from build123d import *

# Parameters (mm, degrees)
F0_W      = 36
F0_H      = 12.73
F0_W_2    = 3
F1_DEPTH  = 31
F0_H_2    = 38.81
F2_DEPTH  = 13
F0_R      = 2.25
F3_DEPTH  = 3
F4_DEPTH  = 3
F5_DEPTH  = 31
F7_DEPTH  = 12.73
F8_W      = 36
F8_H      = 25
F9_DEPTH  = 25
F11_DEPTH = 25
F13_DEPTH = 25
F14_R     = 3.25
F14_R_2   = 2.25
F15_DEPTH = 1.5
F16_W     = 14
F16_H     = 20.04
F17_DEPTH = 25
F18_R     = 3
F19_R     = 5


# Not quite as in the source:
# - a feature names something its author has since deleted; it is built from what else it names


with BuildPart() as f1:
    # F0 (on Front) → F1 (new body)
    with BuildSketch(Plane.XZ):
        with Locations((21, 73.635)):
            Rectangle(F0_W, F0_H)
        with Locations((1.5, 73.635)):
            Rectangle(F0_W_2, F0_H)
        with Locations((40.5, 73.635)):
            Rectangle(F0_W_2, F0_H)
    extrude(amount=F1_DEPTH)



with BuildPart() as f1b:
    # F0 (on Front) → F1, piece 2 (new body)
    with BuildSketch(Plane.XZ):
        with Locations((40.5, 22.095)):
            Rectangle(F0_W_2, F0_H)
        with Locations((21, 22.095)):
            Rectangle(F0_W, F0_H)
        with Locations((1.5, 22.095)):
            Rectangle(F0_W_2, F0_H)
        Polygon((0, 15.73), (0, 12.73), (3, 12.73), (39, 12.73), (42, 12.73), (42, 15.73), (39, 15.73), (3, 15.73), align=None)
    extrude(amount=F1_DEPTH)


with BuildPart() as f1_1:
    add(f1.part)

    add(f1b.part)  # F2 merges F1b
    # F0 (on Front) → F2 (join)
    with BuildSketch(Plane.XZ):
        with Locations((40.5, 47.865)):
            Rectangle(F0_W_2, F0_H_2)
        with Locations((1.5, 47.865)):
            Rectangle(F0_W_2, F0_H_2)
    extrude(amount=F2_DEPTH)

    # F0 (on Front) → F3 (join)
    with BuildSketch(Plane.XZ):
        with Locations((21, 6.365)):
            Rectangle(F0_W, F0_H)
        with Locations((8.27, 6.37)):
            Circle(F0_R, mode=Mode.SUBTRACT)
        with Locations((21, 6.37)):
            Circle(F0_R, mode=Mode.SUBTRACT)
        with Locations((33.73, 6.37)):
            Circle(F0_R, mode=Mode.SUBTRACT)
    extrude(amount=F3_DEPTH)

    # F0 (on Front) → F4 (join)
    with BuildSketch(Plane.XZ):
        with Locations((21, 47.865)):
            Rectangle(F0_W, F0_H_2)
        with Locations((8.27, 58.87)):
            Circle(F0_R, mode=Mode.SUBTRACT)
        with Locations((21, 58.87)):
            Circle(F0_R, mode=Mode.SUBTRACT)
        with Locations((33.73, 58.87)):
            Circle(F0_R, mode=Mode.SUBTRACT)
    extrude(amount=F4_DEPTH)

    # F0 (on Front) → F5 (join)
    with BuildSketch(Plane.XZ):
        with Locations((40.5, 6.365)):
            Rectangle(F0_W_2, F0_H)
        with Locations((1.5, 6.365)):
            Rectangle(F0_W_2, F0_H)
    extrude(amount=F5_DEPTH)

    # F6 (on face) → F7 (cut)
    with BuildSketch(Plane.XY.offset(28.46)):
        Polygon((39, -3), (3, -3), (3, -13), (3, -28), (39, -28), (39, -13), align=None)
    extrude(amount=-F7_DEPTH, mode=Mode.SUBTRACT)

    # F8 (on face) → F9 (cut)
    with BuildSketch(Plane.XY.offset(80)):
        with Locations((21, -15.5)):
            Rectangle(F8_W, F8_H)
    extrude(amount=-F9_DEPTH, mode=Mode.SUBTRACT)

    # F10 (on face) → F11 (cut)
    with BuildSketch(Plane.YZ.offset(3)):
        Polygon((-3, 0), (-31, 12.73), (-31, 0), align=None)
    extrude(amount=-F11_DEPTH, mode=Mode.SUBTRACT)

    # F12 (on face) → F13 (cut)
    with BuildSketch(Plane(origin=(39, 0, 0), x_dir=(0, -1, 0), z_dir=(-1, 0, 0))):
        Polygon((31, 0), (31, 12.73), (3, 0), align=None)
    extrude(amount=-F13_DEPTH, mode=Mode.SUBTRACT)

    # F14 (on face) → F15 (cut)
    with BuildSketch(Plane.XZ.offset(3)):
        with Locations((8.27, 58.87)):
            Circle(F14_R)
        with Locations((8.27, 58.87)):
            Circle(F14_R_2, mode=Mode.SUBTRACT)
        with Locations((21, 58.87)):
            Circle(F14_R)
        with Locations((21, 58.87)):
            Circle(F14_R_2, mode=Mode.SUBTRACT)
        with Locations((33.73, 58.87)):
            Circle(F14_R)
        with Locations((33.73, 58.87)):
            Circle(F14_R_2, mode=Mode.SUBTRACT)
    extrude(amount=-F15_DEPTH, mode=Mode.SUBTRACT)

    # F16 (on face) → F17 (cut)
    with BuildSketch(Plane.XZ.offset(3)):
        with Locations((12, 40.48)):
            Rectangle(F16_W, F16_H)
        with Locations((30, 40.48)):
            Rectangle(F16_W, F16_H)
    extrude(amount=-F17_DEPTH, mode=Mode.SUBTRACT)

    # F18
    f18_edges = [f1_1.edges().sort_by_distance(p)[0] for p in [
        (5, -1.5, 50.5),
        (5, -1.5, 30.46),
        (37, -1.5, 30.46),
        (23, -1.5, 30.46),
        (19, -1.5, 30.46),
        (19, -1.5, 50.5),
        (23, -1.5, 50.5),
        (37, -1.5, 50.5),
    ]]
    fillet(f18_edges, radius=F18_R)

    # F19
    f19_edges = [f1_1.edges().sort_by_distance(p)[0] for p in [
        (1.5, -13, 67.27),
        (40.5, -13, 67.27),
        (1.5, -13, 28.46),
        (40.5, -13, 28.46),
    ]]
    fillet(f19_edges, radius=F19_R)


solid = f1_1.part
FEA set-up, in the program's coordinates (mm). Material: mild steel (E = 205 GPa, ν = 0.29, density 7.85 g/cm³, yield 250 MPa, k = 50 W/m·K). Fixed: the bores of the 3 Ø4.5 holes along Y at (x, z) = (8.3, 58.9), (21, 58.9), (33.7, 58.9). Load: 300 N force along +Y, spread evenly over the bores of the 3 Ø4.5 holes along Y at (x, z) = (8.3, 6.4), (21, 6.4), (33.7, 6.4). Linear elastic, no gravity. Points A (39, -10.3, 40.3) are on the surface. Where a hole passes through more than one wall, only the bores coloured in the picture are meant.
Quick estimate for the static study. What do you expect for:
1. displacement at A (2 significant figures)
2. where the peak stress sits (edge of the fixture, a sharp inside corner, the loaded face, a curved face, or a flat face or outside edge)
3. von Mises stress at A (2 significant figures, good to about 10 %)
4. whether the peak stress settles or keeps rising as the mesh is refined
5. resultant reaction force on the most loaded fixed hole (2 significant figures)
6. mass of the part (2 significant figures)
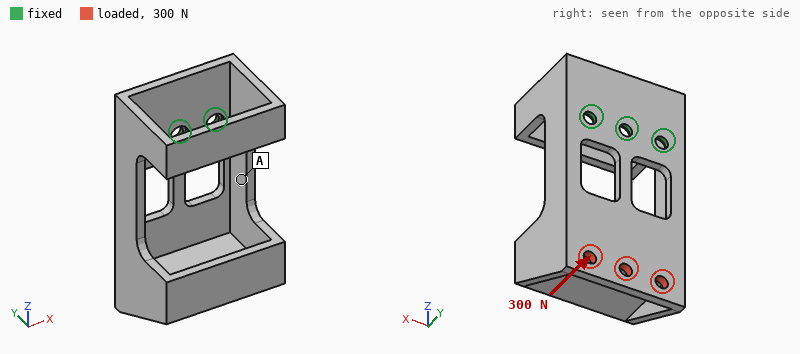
0.088 mm
edge of the fixture
30 MPa
keeps rising
290 N
170 g
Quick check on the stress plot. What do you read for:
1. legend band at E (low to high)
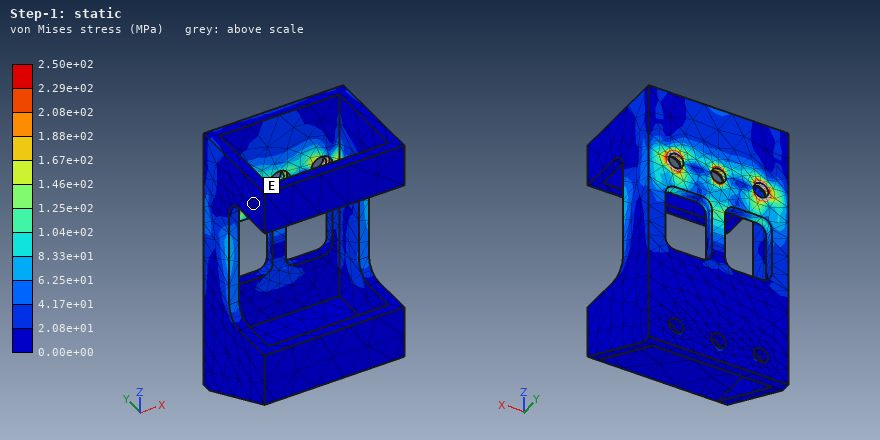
0.00e+00 to 2.08e+01 MPa
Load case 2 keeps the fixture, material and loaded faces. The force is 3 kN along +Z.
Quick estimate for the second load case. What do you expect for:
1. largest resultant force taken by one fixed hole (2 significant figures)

1.1 kN
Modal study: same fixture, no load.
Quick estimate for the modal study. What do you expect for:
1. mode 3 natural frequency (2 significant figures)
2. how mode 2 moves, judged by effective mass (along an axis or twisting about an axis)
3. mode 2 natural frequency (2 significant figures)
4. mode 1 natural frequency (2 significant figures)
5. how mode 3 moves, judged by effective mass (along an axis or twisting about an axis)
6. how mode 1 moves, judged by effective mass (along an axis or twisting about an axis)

2200 Hz
along X
1200 Hz
630 Hz
along X
along Y
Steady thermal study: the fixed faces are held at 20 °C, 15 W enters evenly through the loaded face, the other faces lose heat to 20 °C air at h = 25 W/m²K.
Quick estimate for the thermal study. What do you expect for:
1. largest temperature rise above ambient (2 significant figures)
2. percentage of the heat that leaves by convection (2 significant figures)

69 K
68 %
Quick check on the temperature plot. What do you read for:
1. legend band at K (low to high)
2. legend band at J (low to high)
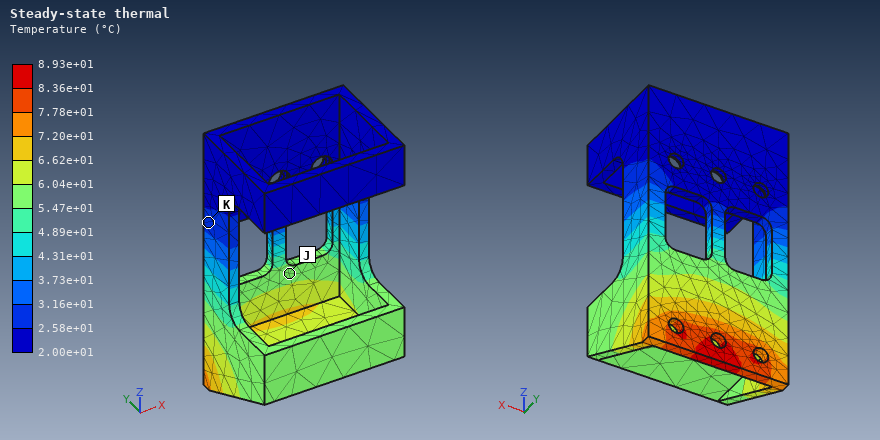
2.58e+01 to 3.16e+01 °C
5.47e+01 to 6.04e+01 °C
